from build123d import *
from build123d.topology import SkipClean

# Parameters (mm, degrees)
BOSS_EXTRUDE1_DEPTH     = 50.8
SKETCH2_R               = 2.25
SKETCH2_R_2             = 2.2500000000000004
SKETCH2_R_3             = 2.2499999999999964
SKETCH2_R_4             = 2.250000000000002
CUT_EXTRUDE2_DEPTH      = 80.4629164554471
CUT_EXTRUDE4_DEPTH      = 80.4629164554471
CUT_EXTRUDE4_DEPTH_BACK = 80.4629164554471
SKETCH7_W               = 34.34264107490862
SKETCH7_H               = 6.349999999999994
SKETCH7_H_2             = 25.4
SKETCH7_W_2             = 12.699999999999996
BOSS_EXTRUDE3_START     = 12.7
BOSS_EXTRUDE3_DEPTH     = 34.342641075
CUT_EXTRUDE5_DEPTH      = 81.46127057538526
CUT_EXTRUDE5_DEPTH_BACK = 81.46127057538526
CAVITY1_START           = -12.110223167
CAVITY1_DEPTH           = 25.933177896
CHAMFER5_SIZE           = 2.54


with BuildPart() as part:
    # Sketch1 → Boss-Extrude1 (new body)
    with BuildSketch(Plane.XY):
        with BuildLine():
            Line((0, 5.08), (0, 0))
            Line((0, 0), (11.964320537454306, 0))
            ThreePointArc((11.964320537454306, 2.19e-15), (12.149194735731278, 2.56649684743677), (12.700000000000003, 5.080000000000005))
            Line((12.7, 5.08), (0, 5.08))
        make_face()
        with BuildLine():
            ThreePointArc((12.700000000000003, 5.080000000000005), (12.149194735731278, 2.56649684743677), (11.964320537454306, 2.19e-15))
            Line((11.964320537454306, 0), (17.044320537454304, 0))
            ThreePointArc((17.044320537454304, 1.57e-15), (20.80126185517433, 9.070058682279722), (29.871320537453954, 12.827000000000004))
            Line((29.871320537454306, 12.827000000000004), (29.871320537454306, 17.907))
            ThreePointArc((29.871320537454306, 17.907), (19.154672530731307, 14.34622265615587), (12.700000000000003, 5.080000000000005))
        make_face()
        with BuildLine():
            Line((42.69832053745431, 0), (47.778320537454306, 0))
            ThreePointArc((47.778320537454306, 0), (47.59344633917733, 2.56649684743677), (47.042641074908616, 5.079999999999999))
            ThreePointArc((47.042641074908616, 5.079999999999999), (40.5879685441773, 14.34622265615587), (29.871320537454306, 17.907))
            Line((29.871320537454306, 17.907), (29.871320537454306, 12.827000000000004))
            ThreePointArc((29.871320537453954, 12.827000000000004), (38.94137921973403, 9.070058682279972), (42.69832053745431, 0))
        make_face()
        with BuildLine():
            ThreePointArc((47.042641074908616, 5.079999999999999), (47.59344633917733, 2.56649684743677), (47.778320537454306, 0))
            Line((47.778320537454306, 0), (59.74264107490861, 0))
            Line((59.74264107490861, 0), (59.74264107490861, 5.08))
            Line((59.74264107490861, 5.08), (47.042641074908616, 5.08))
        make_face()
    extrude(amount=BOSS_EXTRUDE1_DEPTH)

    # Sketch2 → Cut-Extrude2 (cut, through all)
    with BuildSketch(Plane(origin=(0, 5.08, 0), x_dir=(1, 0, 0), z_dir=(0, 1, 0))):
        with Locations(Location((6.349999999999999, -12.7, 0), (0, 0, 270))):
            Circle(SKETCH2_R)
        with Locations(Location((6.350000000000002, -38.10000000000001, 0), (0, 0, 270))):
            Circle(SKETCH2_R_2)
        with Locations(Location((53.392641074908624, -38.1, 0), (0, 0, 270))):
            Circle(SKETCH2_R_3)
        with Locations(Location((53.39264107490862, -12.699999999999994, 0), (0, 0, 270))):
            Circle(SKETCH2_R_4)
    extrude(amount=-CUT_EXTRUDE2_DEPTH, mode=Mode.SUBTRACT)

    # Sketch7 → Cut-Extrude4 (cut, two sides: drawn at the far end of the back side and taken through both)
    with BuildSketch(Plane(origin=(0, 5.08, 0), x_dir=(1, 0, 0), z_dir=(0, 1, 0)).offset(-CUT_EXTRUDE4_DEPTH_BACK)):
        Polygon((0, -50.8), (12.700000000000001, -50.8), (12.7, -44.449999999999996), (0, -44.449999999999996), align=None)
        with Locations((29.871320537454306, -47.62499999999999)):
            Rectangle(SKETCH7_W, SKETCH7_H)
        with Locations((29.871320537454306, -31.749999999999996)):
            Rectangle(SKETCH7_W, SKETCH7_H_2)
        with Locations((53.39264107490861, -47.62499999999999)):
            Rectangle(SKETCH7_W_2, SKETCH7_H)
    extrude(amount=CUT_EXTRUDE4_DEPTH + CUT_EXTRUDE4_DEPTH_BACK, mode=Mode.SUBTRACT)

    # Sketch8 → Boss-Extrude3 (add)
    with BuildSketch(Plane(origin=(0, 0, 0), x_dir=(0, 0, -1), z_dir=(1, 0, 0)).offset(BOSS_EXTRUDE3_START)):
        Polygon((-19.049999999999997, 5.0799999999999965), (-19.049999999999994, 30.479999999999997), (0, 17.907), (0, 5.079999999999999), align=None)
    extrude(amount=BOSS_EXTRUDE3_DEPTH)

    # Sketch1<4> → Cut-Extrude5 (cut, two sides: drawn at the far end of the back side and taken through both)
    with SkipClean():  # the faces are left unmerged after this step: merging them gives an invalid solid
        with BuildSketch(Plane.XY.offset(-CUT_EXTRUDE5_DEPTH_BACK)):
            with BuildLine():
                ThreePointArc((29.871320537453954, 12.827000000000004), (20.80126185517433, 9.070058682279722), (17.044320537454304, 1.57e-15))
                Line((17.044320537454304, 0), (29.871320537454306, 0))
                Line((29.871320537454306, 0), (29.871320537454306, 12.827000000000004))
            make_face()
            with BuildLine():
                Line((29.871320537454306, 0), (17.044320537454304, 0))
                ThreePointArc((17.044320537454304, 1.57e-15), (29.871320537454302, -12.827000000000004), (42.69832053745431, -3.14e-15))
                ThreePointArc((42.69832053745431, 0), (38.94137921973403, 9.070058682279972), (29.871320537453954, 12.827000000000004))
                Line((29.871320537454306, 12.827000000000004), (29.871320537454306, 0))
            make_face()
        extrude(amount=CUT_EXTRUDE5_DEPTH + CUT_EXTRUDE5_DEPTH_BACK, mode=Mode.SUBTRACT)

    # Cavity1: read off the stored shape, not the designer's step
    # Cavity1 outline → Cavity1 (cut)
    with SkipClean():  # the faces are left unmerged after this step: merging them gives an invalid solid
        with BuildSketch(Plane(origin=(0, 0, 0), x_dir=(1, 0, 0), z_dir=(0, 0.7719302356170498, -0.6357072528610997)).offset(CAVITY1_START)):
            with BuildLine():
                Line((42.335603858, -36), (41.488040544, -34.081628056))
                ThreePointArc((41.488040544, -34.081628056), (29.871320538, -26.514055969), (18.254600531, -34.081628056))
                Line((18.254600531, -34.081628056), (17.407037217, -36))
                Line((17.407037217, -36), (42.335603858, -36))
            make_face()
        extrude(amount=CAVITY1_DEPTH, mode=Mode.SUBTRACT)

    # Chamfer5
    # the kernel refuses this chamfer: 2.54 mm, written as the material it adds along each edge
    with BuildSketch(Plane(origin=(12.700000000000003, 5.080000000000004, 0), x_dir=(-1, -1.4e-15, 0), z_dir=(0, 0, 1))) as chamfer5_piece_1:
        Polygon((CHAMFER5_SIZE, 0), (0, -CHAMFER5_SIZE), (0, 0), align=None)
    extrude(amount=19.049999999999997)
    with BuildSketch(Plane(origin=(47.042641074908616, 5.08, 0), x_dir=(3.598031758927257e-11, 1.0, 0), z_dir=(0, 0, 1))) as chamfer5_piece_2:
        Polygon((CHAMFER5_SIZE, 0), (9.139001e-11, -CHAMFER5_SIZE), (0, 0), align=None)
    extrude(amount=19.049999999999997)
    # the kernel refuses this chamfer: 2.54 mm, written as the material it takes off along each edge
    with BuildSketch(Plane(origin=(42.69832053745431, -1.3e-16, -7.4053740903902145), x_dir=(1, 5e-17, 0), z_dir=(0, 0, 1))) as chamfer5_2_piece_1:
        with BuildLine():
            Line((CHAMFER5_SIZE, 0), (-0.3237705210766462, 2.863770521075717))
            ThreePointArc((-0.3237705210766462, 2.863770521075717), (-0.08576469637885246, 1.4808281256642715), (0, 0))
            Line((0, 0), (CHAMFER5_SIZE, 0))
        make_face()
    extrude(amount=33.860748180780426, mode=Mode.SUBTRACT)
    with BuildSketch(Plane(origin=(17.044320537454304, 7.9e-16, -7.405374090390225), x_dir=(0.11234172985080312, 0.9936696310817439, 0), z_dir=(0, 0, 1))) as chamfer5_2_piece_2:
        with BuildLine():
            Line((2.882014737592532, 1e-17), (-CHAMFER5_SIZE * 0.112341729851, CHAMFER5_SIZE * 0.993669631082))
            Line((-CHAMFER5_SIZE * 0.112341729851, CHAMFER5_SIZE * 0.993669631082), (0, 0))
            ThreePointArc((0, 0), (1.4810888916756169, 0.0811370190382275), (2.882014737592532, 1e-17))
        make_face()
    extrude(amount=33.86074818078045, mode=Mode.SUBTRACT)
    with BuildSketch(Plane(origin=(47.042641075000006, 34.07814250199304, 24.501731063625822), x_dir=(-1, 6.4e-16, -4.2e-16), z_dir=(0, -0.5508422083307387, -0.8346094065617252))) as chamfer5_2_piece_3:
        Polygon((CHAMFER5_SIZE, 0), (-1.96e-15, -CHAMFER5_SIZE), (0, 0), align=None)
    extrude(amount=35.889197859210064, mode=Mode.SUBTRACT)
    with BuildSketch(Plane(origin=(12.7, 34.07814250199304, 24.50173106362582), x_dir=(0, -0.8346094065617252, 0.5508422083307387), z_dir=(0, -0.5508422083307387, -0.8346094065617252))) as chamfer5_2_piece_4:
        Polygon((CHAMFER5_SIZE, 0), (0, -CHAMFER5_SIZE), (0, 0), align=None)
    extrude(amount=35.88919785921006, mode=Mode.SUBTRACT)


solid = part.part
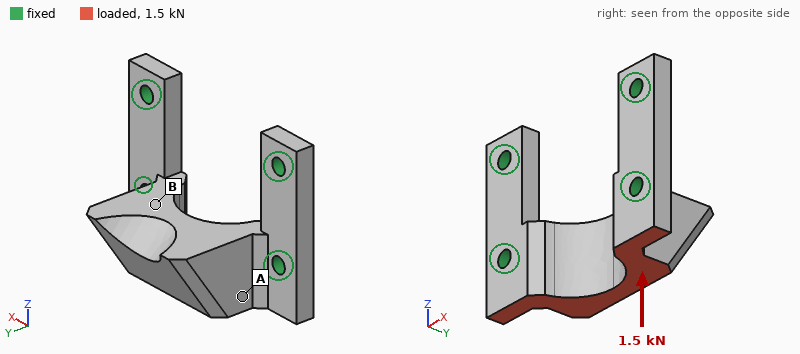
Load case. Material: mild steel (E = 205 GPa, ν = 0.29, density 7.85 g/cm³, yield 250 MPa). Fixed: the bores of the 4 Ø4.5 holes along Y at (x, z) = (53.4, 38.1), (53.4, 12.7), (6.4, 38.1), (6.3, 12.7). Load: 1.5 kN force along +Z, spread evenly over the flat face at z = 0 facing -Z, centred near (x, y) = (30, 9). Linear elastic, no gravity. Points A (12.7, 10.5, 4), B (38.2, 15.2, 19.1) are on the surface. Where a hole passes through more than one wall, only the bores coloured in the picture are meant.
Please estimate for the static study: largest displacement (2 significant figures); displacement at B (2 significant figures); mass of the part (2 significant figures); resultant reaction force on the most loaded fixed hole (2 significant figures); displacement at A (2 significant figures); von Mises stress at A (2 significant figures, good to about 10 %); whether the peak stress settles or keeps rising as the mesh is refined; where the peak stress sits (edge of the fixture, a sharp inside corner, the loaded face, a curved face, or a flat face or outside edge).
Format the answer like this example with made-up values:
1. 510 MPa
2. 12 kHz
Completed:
1. 14 µm
2. 7.4 µm
3. 120 g
4. 640 N
5. 5.9 µm
6. 12 MPa
7. keeps rising
8. edge of the fixture
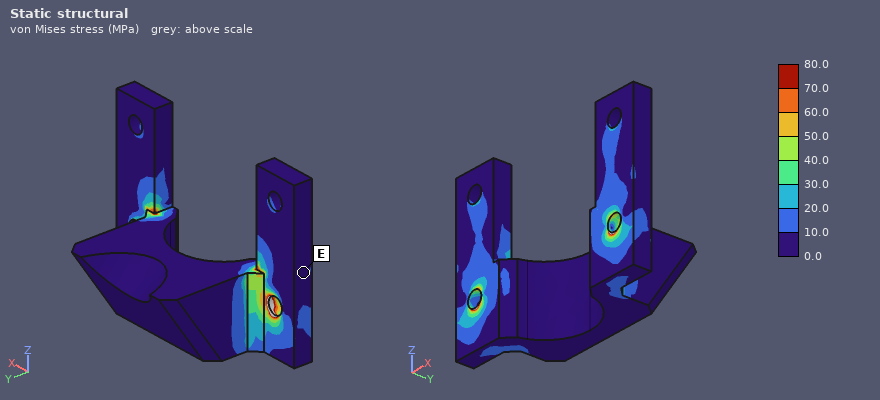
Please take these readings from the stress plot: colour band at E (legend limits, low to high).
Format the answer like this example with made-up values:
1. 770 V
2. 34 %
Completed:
1. 0.0 to 10.0 MPa
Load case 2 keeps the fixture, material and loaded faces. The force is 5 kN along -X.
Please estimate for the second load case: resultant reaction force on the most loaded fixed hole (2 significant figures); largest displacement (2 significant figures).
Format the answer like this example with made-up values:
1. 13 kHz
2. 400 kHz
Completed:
1. 2.8 kN
2. 10 µm
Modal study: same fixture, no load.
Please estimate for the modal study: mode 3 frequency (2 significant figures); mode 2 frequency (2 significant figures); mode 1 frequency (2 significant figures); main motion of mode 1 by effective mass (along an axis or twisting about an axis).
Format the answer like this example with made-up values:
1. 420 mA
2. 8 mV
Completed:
1. 16 kHz
2. 15 kHz
3. 5300 Hz
4. along Z
